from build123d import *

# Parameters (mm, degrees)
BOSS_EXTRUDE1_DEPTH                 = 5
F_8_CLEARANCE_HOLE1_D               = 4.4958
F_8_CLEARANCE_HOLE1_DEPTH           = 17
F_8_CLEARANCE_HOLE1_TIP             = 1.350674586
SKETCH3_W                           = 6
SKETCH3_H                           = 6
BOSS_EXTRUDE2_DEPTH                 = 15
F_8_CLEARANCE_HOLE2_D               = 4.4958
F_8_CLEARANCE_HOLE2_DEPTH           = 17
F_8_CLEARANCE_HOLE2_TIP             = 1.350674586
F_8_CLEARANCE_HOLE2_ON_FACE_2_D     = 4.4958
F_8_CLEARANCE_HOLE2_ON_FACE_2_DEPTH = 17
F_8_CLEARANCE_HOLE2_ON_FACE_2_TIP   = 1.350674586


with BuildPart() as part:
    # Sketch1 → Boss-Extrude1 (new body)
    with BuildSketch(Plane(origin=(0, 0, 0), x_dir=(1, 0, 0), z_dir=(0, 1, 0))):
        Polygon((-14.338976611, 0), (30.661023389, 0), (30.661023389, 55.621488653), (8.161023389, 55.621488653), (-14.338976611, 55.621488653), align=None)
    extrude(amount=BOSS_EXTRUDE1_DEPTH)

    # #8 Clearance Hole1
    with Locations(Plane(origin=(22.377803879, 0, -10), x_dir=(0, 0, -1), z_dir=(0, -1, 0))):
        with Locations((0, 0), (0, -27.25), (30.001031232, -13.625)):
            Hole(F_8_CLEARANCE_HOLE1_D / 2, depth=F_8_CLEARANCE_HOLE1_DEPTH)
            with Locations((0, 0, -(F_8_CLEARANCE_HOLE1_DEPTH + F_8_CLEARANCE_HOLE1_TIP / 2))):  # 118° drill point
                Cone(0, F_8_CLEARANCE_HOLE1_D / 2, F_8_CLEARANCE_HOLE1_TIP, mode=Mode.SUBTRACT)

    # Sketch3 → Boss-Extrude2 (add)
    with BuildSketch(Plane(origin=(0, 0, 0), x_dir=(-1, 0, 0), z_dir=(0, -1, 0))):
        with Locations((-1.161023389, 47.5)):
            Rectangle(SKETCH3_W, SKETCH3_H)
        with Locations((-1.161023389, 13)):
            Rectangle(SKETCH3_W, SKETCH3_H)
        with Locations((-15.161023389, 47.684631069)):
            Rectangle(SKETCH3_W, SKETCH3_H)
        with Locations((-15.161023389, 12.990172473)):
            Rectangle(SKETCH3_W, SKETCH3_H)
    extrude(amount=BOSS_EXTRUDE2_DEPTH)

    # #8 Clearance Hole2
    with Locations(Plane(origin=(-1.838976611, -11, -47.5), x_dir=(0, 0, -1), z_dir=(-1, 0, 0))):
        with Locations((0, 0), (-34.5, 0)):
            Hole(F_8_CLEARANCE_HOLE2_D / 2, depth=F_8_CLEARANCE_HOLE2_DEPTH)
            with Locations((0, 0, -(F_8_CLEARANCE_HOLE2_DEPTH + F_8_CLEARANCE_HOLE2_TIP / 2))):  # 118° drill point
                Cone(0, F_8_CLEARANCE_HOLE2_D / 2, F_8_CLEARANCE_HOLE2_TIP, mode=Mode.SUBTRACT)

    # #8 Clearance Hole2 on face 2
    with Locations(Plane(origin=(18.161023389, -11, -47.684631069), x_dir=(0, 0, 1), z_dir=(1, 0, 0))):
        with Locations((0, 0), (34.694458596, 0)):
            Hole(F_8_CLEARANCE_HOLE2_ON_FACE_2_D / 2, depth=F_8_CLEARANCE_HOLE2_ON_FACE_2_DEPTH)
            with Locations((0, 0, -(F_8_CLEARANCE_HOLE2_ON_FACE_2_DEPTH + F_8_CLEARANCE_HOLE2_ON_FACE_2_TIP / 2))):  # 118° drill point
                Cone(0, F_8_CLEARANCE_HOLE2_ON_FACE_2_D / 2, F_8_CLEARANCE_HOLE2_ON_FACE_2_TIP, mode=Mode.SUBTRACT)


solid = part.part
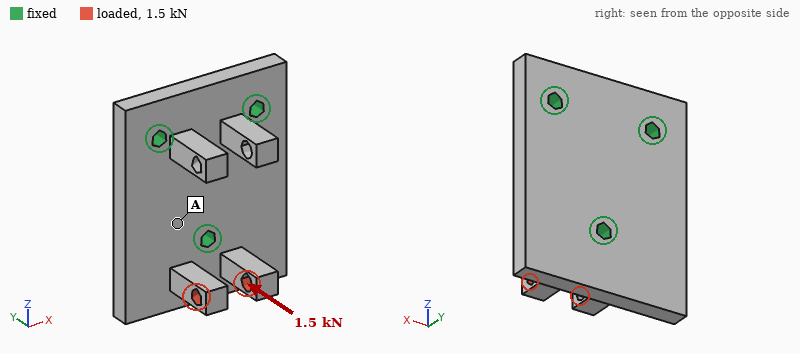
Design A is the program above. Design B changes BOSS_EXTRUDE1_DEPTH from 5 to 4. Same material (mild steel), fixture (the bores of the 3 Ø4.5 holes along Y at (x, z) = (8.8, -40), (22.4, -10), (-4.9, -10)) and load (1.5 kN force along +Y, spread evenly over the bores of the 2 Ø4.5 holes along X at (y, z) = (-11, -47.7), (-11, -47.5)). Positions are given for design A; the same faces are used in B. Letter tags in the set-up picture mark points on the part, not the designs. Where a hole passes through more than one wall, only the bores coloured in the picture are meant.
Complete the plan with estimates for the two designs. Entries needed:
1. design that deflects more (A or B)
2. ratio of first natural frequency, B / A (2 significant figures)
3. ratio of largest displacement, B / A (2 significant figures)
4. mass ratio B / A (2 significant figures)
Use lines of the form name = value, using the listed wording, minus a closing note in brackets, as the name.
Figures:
design that deflects more = B
ratio of first natural frequency, B / A = 0.82
ratio of largest displacement, B / A = 1.7
mass ratio B / A = 0.83
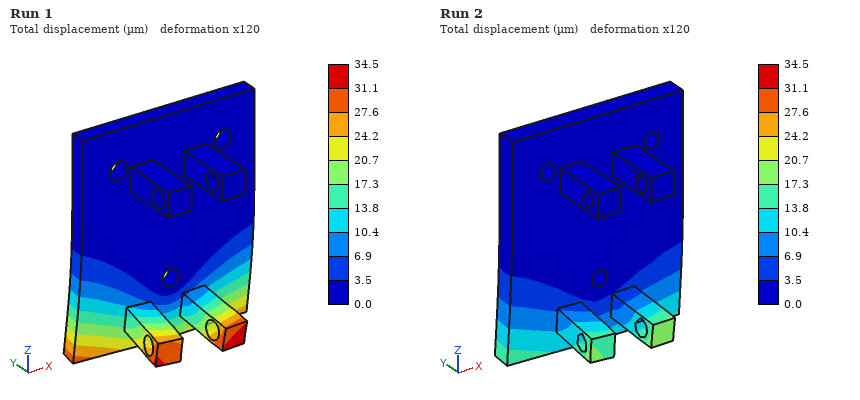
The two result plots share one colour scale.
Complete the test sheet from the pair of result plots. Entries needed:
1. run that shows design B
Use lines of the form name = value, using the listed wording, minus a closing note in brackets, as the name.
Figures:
run that shows design B = Run 1
